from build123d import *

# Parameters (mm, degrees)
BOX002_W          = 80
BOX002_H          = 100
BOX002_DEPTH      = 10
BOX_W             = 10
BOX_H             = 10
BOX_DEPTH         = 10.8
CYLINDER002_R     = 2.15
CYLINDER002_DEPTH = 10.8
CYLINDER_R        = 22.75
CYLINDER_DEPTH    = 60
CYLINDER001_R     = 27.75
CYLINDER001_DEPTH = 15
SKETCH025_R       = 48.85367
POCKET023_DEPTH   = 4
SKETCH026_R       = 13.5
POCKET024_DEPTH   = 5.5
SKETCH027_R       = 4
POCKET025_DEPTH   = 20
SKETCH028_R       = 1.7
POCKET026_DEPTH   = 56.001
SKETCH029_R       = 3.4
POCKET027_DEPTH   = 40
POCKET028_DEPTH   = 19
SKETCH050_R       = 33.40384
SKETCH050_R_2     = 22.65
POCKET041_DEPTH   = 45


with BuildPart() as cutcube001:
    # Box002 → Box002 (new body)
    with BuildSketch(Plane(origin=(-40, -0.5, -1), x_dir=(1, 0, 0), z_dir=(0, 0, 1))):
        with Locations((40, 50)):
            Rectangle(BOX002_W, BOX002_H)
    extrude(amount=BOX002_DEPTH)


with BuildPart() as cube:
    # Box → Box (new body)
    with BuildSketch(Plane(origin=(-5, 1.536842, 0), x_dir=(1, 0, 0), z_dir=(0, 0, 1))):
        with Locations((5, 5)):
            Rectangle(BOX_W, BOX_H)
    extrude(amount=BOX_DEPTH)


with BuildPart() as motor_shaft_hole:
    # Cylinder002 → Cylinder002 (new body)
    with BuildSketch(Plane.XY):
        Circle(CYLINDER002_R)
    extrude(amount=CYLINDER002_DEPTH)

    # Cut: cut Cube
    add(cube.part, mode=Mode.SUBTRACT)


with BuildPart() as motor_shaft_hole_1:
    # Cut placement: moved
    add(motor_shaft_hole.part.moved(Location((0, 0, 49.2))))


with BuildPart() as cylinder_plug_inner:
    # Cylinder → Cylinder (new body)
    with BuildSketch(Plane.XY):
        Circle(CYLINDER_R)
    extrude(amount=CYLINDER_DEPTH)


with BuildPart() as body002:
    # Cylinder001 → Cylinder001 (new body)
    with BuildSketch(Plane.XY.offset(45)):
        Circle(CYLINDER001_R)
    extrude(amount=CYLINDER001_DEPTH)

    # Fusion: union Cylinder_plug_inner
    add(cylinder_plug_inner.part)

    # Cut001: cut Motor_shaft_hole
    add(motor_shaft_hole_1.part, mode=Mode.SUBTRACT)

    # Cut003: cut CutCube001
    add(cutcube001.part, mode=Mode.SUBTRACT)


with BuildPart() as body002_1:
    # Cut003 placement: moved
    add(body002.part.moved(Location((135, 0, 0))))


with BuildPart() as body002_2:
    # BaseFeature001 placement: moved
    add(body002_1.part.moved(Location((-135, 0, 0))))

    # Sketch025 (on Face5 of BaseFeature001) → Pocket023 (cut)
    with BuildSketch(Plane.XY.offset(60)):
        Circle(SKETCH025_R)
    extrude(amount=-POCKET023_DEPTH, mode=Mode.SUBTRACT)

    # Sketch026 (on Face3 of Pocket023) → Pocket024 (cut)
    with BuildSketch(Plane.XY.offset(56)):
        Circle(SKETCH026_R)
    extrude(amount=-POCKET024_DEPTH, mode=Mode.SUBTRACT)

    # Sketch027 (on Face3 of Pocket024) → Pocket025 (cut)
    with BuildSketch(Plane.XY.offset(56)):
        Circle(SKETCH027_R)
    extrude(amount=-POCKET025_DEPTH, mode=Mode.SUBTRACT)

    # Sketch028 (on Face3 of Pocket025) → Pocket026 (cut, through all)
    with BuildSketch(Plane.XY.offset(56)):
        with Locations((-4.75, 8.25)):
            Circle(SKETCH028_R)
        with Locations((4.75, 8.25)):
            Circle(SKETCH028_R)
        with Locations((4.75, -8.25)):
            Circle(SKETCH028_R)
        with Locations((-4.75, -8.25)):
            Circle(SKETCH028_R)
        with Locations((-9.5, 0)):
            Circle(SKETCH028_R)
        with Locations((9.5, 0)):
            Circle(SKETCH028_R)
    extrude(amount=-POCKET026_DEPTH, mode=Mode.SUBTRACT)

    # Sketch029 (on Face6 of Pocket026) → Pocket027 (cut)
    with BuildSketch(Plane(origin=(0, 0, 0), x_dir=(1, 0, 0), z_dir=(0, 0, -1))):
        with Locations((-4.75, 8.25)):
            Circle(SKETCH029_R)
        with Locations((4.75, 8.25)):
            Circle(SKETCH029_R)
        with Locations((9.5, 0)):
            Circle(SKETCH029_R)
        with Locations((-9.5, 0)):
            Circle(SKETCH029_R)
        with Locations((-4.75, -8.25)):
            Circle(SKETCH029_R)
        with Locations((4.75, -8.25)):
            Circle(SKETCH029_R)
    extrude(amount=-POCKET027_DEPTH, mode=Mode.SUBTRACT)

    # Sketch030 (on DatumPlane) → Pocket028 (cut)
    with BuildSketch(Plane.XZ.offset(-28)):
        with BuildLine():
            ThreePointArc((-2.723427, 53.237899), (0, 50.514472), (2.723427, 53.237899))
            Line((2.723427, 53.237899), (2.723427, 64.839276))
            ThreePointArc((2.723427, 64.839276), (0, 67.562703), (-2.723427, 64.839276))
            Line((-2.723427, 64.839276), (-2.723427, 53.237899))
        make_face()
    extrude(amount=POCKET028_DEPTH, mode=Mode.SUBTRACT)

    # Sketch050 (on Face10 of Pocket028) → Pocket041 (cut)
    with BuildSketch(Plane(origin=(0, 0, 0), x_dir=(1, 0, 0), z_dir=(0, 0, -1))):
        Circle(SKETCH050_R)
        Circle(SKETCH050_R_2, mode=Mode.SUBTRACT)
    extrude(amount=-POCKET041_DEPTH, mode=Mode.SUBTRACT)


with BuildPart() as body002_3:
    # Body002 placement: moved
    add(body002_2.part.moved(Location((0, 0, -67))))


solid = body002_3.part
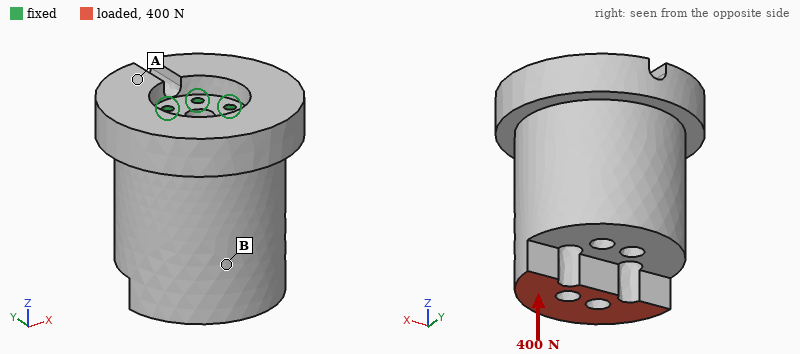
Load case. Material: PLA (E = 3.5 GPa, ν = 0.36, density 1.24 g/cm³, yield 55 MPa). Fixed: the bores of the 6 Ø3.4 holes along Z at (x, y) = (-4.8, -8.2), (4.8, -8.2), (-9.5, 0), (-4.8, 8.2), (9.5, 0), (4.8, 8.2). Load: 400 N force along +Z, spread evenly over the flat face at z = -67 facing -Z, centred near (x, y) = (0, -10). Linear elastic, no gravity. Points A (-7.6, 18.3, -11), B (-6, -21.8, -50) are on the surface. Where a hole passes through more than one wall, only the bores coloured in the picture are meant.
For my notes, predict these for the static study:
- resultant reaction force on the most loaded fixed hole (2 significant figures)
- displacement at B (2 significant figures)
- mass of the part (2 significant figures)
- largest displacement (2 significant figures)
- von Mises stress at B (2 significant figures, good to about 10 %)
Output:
150 N
16 µm
98 g
23 µm
0.69 MPa
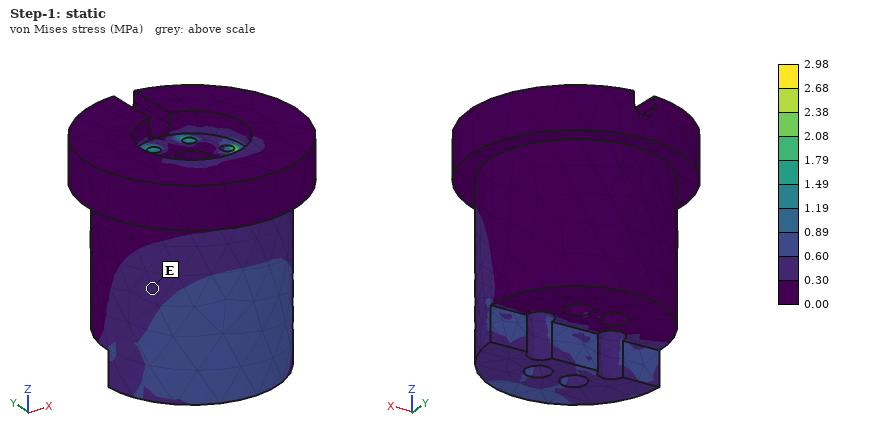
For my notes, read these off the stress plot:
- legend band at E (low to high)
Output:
0.30 to 0.60 MPa
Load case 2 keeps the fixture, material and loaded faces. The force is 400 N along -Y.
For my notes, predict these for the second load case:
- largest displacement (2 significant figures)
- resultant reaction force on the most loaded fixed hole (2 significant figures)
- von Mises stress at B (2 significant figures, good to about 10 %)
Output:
0.10 mm
340 N
1.7 MPa
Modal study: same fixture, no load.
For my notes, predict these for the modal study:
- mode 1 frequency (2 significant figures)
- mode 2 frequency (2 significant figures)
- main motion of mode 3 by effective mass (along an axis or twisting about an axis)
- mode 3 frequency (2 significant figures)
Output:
2300 Hz
2300 Hz
twisting about Z
4500 Hz
